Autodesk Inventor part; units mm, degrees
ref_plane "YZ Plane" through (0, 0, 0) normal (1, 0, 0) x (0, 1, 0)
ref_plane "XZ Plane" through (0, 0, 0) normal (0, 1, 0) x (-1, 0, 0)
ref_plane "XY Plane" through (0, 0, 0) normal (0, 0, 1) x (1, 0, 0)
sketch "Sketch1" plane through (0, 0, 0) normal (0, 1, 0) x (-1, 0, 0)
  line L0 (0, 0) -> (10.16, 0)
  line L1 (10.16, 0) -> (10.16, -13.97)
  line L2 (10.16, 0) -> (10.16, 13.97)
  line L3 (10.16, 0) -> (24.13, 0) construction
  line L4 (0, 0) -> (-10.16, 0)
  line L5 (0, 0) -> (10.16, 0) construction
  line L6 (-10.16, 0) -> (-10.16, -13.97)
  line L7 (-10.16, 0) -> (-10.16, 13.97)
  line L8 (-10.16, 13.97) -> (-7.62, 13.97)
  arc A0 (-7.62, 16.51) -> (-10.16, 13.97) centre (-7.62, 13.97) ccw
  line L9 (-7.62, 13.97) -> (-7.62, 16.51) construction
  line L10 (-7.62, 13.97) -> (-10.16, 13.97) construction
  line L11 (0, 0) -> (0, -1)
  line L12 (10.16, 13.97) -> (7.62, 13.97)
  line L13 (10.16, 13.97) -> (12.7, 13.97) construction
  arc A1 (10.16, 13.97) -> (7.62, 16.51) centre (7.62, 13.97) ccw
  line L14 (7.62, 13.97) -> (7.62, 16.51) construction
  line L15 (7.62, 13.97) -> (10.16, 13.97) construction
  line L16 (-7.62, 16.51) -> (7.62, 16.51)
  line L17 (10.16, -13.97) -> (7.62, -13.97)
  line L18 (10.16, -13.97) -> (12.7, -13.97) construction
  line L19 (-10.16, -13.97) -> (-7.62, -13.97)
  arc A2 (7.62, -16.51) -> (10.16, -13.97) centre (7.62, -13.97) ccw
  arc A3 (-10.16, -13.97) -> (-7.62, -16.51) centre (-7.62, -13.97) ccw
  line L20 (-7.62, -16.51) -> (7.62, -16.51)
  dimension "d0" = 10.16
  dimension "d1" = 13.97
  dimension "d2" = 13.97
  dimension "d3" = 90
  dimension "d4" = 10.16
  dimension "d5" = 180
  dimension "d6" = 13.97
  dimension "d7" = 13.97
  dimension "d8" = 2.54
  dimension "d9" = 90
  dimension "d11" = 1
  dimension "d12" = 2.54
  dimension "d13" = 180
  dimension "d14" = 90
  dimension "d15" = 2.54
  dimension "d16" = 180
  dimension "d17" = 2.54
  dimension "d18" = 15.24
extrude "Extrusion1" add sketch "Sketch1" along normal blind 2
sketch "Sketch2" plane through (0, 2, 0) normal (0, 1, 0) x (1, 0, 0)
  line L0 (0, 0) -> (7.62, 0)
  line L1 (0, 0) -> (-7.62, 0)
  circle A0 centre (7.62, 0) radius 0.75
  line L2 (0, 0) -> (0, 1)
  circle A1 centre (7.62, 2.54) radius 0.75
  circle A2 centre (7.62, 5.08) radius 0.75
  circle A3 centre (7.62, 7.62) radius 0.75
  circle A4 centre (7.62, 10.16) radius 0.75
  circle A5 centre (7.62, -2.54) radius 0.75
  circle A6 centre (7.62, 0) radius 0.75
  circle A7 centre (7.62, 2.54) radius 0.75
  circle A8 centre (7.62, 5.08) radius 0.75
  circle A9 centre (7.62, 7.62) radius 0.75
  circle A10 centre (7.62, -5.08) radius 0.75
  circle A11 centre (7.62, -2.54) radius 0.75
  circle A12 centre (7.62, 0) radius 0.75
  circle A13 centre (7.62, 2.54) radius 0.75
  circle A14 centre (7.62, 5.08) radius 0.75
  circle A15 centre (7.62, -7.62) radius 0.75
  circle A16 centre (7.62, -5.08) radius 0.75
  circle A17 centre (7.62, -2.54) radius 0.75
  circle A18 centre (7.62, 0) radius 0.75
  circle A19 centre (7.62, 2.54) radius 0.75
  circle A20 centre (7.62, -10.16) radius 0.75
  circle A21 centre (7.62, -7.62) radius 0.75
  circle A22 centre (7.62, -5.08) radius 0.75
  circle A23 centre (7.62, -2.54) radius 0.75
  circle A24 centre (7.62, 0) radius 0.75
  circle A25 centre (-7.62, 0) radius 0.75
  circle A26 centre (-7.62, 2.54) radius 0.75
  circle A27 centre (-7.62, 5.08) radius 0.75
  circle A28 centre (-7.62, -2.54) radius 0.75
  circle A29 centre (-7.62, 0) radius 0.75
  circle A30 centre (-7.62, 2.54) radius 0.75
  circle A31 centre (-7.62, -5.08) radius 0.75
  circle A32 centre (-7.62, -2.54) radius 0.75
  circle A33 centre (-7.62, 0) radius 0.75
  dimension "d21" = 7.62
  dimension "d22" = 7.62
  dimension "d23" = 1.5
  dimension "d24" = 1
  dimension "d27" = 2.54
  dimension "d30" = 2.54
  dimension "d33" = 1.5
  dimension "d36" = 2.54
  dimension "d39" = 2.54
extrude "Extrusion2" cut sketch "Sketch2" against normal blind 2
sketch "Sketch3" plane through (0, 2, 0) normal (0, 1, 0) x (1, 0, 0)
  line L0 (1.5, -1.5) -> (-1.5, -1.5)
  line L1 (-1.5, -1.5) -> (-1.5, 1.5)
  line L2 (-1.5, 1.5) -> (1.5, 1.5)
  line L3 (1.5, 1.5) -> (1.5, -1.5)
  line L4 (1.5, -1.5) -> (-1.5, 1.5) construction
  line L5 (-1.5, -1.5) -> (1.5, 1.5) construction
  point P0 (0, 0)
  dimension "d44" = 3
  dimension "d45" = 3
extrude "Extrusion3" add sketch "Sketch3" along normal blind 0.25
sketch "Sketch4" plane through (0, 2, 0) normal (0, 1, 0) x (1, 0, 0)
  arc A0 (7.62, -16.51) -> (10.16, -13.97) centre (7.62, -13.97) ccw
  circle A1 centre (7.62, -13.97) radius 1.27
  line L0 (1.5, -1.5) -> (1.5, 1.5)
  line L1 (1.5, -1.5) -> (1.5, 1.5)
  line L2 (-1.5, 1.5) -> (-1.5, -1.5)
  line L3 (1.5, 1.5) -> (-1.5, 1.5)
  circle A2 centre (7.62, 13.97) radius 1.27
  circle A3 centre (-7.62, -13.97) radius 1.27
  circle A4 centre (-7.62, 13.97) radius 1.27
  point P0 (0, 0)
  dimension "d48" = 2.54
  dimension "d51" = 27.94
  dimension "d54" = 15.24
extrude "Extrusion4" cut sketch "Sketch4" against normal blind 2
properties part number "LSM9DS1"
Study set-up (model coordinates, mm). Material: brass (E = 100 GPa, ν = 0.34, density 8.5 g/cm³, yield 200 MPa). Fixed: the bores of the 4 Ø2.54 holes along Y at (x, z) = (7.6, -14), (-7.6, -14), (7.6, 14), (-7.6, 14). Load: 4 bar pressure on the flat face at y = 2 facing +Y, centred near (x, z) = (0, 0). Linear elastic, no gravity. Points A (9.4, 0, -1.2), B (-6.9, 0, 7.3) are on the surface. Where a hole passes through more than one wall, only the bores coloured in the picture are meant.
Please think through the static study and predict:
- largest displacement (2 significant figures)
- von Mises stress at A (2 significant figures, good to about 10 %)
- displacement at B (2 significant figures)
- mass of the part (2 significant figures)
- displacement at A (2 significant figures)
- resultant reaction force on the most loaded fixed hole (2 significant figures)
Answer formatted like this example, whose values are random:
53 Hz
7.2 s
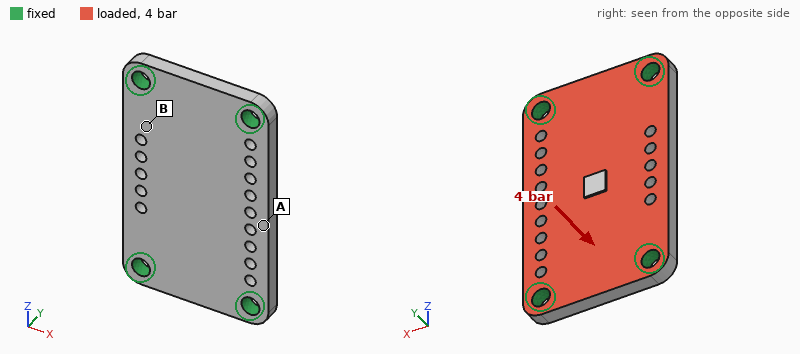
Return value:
10 µm
22 MPa
5.1 µm
11 g
9.9 µm
62 N
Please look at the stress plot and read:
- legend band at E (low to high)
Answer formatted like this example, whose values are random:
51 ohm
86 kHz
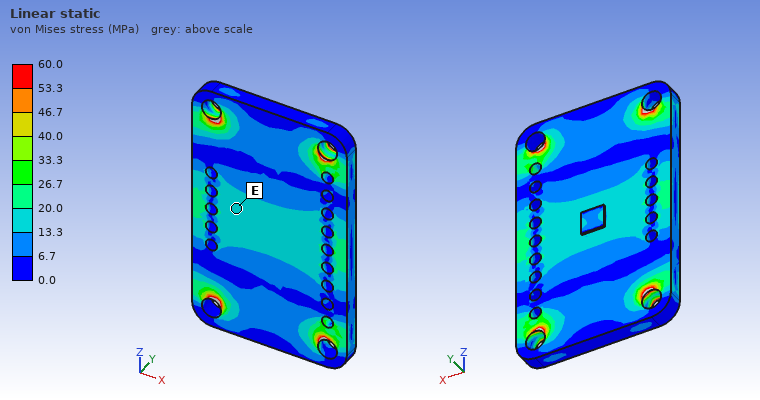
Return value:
13.3 to 20.0 MPa
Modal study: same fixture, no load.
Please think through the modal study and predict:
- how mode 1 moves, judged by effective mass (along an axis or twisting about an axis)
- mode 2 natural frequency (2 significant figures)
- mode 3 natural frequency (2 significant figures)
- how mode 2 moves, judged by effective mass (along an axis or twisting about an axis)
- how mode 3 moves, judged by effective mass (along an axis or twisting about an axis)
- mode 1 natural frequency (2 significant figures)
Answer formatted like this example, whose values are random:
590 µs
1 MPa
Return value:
along Y
13 kHz
22 kHz
twisting about Z
twisting about X
8700 Hz
